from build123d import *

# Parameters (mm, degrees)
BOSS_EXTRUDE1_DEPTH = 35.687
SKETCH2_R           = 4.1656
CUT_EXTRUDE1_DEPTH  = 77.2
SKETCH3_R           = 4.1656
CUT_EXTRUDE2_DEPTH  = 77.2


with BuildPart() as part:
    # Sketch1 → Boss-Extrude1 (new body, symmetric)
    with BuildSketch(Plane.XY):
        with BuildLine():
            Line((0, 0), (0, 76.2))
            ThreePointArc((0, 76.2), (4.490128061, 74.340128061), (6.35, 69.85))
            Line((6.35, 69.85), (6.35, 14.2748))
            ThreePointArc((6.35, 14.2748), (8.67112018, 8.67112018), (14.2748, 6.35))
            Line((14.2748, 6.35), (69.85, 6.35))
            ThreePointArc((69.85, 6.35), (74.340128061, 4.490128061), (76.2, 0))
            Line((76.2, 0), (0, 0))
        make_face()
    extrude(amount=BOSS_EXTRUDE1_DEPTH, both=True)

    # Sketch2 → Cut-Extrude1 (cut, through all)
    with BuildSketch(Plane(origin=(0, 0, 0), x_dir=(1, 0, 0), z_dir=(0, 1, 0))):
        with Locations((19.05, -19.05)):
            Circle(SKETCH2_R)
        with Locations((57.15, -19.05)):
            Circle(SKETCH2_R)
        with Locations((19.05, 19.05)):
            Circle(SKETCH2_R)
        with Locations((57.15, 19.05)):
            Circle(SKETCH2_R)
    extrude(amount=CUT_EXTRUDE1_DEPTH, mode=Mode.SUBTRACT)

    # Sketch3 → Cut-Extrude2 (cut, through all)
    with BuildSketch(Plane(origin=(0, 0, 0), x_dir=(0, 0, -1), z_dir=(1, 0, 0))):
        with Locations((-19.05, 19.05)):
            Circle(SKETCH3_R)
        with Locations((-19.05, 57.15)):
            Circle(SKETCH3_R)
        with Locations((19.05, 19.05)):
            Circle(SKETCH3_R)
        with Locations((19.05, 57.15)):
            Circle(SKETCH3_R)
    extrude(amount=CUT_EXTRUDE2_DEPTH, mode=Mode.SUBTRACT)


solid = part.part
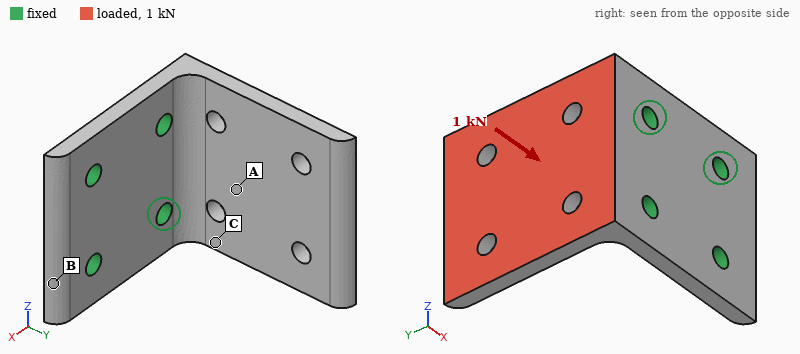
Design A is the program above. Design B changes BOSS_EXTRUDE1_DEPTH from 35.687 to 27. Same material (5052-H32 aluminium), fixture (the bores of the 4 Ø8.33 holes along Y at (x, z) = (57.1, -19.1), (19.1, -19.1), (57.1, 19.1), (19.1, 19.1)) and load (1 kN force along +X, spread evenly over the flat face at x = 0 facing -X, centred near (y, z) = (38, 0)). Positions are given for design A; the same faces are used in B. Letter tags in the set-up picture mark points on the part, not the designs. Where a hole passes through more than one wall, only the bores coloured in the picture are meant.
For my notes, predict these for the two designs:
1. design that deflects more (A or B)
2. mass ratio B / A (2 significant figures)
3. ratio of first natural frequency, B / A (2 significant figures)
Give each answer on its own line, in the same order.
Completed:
B
0.75
1.0
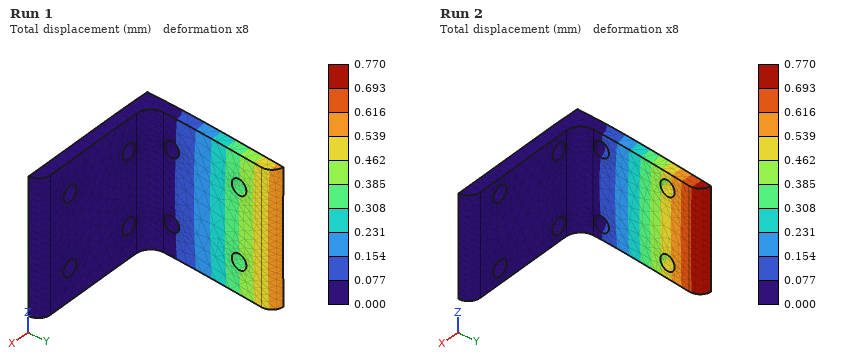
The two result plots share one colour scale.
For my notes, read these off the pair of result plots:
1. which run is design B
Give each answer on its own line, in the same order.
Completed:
Run 2
